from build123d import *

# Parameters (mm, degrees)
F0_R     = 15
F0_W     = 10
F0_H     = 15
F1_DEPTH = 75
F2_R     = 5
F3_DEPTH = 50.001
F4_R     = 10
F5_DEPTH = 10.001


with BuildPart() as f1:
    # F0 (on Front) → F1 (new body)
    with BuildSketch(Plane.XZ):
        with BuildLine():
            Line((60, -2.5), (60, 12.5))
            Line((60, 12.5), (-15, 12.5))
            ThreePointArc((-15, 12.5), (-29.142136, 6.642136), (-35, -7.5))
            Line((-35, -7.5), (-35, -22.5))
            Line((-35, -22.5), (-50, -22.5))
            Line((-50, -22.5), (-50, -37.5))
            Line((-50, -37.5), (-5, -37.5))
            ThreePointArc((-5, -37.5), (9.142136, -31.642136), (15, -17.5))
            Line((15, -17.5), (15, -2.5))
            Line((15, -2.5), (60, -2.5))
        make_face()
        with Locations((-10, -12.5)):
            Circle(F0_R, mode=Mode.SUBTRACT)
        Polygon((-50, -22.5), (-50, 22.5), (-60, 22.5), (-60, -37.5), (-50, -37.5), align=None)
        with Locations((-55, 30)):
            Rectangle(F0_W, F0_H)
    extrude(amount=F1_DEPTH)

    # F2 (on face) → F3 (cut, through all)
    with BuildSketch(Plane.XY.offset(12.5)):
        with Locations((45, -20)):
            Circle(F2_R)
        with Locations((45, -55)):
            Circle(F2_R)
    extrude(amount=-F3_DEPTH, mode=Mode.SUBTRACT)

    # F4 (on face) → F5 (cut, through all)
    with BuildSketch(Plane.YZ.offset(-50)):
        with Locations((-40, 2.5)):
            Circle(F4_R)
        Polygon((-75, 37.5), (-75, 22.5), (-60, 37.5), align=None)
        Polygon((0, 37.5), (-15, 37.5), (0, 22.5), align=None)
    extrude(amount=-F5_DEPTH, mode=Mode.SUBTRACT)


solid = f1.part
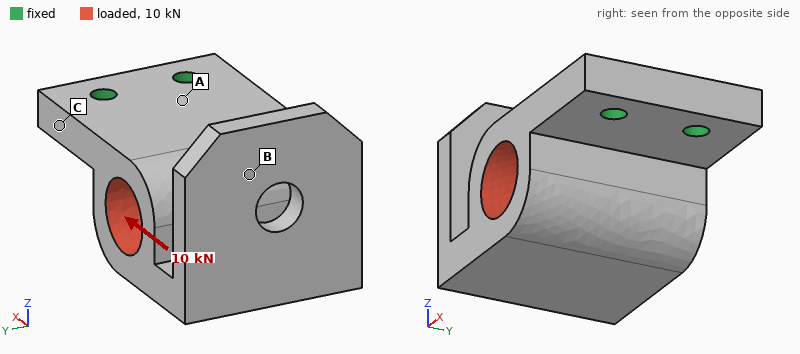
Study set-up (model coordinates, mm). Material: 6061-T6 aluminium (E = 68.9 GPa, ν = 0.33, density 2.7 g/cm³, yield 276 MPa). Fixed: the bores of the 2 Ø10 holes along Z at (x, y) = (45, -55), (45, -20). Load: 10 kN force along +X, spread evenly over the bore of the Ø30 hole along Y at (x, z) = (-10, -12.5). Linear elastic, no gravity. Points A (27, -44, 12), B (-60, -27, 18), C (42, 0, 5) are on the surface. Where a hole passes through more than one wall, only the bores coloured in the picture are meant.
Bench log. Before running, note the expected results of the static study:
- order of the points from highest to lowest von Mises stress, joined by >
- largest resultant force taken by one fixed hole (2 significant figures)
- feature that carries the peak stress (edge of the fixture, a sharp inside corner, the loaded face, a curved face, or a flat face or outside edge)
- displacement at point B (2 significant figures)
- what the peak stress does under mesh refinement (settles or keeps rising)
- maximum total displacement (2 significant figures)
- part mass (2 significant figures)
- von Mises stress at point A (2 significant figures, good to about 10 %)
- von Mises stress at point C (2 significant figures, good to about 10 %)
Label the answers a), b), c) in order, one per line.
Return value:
a) A > C > B
b) 5.0 kN
c) edge of the fixture
d) 0.40 mm
e) keeps rising
f) 0.45 mm
g) 640 g
h) 47 MPa
i) 19 MPa
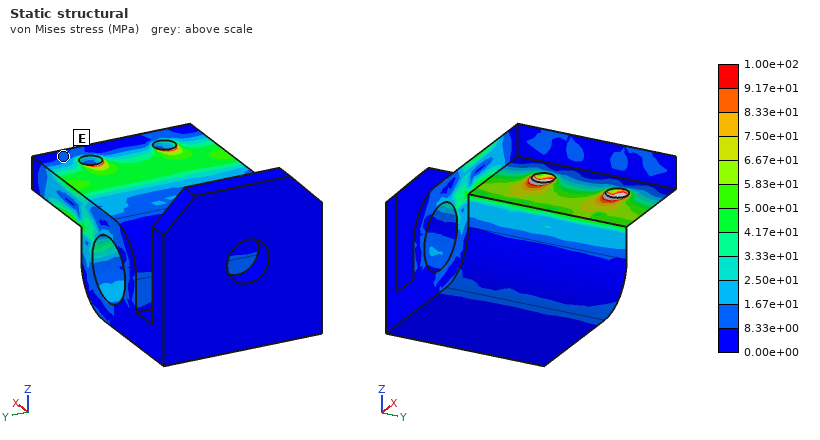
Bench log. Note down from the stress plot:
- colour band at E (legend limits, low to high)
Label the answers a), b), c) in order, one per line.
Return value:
a) 8.33e+00 to 1.67e+01 MPa
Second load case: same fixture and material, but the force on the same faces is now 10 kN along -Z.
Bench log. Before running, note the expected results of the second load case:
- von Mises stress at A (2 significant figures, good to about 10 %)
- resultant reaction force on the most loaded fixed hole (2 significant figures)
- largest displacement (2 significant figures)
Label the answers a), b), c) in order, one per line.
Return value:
a) 120 MPa
b) 5.0 kN
c) 0.95 mm
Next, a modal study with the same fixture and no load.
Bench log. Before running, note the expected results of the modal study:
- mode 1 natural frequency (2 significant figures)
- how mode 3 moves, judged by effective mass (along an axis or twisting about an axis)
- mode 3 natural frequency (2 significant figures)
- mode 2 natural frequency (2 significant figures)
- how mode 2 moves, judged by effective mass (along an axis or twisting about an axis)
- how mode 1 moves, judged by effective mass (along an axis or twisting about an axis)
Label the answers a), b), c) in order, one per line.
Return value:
a) 680 Hz
b) along Y
c) 1900 Hz
d) 1700 Hz
e) along X
f) along Z
